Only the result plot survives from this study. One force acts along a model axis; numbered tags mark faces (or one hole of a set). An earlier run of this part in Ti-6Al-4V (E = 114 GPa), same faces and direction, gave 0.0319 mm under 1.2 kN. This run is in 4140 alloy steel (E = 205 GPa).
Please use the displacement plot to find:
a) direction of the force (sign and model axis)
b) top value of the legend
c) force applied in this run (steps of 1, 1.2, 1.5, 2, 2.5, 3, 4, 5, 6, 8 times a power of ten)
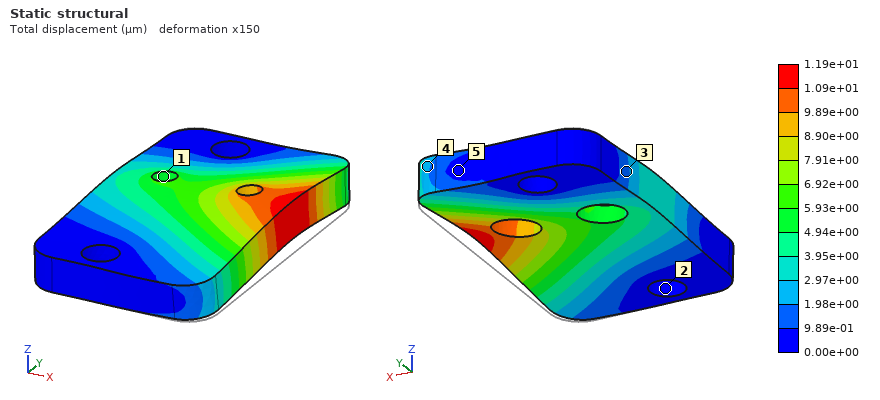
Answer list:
+Z
1.19e+01 µm
800 N
